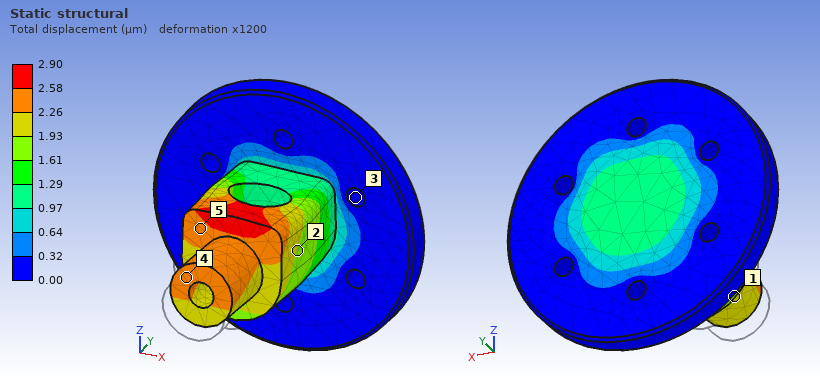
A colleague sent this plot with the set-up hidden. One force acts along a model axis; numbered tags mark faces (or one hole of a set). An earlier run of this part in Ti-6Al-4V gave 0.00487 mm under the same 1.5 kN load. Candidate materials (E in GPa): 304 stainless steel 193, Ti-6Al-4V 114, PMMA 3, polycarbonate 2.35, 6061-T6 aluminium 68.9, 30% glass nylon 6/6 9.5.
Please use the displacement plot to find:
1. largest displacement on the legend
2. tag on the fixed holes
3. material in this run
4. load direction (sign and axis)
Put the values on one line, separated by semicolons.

2.90 µm; 3; 304 stainless steel; +Y
